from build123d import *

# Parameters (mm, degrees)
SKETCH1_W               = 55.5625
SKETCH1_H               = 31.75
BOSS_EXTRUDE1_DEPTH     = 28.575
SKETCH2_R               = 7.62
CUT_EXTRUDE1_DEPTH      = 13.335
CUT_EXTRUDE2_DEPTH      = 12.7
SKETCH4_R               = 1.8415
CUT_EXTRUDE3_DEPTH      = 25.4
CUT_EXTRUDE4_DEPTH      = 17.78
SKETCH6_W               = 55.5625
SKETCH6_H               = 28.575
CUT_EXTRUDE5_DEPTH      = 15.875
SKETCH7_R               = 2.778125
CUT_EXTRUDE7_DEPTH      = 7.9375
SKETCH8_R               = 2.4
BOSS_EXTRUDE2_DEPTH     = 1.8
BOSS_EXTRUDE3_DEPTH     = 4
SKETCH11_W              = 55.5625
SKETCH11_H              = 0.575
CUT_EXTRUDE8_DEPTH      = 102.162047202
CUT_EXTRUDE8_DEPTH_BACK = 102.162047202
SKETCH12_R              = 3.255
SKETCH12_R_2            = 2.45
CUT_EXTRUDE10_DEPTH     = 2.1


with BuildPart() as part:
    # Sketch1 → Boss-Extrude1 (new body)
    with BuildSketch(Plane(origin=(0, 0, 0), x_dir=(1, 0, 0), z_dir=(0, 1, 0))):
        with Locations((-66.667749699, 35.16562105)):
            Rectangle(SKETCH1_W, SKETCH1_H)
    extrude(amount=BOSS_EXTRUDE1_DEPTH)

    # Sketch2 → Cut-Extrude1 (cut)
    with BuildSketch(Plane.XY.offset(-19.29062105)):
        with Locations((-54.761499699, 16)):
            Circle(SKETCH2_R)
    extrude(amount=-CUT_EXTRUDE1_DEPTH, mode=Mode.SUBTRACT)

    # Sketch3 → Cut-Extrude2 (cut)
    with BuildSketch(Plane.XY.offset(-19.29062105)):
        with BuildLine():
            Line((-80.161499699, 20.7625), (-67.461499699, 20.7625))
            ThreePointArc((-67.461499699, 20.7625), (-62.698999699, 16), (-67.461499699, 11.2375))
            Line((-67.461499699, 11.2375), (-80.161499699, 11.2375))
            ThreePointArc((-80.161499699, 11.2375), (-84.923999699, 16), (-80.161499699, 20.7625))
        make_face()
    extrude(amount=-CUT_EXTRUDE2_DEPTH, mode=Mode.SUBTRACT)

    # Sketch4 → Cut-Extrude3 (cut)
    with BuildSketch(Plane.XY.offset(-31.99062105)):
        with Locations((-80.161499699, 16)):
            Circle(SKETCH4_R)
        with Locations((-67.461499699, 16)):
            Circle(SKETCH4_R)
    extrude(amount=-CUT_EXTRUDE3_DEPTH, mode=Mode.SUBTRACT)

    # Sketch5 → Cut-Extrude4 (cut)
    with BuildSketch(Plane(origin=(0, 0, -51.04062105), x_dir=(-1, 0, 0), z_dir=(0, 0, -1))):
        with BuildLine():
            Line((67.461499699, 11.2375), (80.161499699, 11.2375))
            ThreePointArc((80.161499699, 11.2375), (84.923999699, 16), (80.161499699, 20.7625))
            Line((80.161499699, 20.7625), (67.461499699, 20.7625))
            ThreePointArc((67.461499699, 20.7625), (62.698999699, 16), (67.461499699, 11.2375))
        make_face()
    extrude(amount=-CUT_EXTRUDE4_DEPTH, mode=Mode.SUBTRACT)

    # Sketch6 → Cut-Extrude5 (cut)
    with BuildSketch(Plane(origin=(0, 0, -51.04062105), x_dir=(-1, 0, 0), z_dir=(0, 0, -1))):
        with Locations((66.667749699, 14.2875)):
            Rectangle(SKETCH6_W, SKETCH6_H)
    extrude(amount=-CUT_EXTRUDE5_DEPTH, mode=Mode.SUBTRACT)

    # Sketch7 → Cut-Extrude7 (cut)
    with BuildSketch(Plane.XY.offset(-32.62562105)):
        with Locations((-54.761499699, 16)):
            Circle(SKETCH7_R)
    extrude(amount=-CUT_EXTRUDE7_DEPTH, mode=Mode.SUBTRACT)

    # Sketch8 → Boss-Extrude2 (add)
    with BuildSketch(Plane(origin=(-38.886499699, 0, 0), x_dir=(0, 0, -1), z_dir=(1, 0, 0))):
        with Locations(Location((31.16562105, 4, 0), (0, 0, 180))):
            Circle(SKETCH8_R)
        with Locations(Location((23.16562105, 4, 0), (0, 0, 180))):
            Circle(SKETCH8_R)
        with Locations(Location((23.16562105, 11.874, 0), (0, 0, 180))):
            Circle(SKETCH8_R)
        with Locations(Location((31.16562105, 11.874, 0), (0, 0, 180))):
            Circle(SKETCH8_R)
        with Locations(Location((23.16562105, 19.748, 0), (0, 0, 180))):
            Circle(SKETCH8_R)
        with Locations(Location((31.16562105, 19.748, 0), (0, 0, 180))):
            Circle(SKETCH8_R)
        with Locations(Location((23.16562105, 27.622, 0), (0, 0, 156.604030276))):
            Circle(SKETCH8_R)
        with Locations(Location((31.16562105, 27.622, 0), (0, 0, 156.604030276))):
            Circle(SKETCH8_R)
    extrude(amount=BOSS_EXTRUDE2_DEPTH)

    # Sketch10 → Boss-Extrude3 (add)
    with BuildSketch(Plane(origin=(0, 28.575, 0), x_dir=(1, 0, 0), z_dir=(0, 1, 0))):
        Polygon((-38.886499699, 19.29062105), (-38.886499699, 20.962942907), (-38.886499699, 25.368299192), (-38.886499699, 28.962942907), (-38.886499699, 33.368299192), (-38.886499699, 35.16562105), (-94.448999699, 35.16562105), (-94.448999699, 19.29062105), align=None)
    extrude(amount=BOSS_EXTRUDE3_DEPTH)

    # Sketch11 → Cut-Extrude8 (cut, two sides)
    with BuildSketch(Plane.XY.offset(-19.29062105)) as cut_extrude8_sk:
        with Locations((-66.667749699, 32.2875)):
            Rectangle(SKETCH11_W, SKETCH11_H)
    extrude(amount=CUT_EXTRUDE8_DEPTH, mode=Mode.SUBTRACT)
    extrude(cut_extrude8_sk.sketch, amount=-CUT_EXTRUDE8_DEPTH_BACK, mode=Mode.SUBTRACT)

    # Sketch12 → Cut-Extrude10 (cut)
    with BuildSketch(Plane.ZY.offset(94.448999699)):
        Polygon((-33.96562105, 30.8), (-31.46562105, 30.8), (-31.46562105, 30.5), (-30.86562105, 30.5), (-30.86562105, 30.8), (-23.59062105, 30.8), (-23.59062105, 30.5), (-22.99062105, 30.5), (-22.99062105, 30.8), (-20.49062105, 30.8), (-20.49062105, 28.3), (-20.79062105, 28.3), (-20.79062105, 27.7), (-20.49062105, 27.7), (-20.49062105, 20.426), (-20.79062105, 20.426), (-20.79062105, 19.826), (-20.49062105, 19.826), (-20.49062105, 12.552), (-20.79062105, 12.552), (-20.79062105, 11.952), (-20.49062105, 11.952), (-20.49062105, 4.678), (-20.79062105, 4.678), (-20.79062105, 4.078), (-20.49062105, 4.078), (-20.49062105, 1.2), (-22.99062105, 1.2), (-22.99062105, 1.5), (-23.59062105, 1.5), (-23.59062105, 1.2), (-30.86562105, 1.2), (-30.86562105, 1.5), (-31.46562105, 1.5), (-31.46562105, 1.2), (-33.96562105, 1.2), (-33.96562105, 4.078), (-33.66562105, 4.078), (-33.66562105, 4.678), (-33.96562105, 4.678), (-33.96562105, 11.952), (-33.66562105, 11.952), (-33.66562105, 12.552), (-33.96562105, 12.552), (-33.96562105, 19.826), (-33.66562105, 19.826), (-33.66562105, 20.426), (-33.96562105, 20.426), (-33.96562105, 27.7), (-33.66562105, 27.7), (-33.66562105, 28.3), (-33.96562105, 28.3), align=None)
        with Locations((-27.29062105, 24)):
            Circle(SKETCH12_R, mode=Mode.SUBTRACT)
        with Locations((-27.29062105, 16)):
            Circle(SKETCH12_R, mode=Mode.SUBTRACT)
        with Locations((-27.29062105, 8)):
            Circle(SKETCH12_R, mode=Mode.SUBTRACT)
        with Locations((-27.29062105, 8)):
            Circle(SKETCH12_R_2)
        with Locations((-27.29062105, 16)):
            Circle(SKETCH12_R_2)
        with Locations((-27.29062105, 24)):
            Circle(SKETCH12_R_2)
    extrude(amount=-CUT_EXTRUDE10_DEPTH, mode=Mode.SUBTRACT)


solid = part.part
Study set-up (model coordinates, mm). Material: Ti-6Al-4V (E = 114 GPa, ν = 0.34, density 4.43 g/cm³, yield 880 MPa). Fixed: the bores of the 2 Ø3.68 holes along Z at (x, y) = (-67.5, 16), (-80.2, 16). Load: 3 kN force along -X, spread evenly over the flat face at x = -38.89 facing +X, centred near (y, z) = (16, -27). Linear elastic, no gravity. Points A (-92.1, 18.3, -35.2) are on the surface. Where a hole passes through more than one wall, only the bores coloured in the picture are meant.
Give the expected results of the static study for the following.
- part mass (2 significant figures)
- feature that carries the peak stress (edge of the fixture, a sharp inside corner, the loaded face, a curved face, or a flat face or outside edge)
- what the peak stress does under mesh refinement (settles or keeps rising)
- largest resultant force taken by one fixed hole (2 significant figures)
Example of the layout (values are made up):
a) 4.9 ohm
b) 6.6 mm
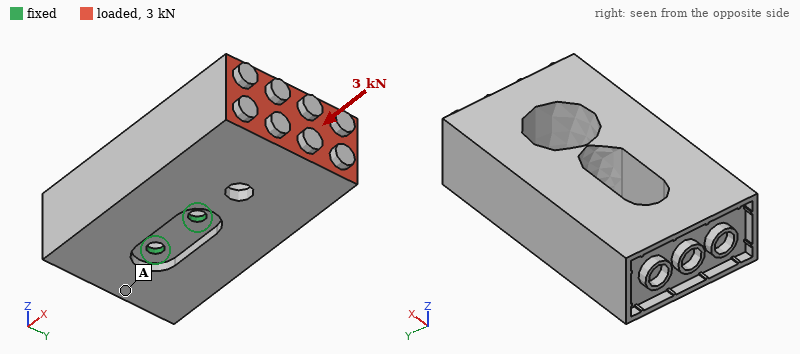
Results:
a) 99 g
b) edge of the fixture
c) keeps rising
d) 1.9 kN
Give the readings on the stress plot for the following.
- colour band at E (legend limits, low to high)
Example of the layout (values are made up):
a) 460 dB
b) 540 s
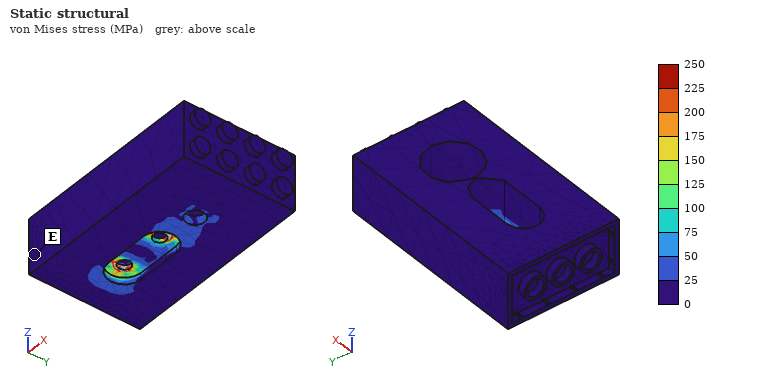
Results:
a) 0 to 25 MPa
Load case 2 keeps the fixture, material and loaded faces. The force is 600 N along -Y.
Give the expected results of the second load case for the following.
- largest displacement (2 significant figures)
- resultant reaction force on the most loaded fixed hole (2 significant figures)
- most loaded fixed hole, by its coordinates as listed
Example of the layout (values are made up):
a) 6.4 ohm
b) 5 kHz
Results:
a) 75 µm
b) 1.7 kN
c) (-67.5, 16)
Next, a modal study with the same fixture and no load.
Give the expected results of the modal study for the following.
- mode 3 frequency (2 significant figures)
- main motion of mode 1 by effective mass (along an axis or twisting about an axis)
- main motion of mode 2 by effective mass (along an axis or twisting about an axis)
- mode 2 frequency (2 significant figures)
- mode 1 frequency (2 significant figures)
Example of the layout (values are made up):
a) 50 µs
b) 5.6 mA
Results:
a) 4500 Hz
b) along Y
c) along Z
d) 2300 Hz
e) 1500 Hz
